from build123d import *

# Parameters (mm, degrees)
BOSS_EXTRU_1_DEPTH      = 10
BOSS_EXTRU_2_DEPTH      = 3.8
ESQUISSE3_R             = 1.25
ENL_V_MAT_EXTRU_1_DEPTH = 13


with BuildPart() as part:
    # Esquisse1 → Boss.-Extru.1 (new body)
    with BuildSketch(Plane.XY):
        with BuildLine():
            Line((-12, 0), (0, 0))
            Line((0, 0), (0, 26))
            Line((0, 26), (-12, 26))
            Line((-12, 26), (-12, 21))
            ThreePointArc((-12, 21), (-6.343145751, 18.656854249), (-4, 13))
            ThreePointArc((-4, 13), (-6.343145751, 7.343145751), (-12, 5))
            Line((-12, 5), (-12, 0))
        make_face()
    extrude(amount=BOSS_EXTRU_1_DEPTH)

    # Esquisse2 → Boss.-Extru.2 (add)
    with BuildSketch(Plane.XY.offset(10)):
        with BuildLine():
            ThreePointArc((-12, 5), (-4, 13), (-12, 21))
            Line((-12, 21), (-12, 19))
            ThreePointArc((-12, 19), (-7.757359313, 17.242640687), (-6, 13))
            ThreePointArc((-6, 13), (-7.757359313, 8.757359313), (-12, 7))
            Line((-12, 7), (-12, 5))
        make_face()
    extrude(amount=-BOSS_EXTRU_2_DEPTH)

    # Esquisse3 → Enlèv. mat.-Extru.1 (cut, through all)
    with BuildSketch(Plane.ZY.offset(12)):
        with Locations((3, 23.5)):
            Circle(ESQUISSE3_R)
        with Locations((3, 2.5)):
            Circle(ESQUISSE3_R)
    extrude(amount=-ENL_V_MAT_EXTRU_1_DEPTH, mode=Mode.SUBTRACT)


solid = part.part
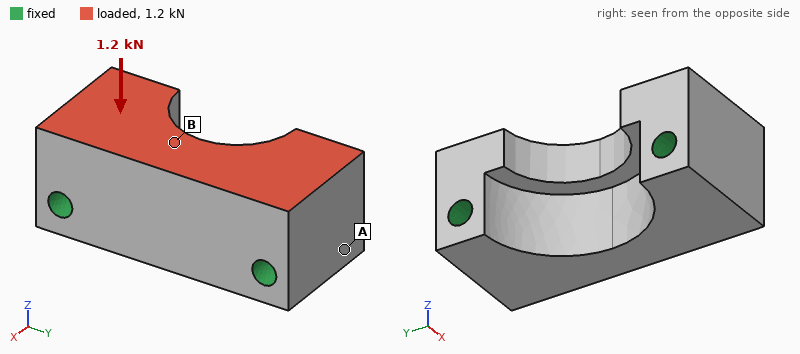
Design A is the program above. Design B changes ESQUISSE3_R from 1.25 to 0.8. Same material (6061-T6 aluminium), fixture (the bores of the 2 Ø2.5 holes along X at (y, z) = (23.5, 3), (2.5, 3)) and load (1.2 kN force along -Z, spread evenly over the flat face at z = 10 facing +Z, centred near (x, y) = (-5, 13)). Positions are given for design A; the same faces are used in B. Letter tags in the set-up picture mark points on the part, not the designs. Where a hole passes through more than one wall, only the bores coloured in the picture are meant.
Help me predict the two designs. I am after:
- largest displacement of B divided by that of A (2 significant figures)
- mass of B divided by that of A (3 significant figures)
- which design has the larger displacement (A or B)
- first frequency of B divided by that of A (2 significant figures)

1.2
1.03
B
0.88
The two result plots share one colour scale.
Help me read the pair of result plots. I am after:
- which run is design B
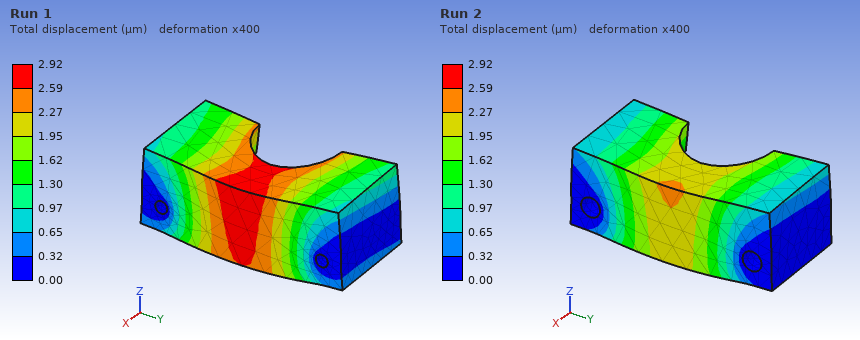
Run 1
